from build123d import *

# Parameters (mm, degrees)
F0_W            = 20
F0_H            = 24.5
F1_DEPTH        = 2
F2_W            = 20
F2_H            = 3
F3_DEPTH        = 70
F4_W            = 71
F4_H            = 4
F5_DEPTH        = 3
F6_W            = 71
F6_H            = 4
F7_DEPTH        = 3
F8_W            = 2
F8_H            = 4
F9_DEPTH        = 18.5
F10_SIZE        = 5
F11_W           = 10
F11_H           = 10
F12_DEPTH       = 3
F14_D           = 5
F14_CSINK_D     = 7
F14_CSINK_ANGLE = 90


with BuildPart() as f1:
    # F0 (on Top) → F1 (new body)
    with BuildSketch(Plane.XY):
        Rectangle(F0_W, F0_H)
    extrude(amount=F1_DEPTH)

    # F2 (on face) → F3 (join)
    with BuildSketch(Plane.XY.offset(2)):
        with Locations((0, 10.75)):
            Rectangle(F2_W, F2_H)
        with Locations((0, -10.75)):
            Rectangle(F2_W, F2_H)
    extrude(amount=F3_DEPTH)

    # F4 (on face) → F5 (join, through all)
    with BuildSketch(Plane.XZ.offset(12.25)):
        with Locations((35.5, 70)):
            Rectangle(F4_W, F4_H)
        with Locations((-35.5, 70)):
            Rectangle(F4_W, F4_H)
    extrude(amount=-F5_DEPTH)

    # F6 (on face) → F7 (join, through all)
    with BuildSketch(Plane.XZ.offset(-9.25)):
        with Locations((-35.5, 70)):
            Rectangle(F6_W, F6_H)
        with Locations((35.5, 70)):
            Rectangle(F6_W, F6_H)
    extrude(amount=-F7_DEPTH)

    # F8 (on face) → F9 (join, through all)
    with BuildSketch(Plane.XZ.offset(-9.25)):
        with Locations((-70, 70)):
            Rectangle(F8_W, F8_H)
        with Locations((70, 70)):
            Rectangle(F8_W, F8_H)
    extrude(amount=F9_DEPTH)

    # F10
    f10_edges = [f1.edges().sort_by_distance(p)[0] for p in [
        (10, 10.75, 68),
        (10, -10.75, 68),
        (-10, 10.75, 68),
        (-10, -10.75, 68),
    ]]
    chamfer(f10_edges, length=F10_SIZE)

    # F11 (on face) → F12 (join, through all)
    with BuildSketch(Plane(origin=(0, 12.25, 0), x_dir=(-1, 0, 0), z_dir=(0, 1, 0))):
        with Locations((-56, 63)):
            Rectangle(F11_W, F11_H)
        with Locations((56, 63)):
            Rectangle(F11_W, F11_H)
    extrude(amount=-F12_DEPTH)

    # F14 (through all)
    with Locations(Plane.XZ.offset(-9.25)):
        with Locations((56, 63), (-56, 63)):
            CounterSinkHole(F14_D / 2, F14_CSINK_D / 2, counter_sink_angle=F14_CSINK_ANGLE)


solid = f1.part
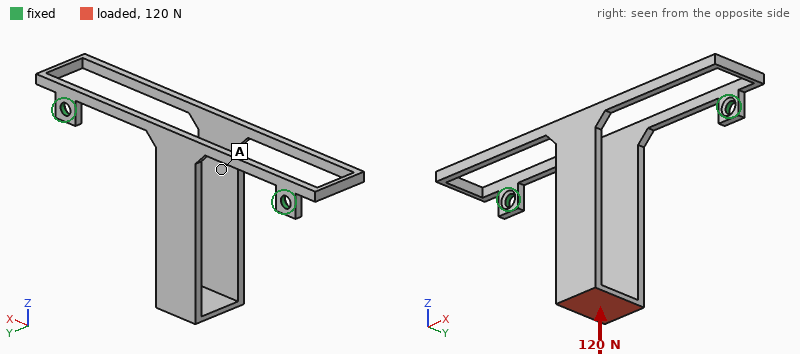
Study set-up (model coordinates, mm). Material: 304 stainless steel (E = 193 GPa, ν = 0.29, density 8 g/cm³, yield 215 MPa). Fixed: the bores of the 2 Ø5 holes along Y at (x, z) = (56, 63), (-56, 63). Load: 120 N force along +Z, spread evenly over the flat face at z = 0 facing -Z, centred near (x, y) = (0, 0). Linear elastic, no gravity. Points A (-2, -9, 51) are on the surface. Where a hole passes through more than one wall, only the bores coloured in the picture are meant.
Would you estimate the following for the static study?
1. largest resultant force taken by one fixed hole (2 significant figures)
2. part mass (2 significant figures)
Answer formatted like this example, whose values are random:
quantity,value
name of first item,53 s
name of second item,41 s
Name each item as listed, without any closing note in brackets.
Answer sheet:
quantity,value
largest resultant force taken by one fixed hole,60 N
part mass,110 g
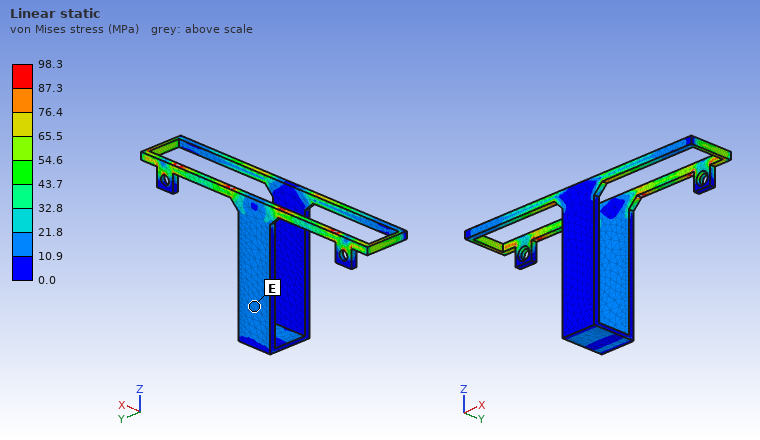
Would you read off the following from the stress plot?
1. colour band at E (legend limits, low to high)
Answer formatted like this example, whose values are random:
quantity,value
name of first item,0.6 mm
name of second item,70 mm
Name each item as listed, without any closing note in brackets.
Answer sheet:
quantity,value
colour band at E,10.9 to 21.8 MPa
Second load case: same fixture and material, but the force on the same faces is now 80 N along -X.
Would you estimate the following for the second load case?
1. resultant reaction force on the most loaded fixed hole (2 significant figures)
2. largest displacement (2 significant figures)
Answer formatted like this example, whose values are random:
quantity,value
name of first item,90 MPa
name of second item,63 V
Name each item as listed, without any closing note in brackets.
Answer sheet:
quantity,value
resultant reaction force on the most loaded fixed hole,78 N
largest displacement,0.29 mm
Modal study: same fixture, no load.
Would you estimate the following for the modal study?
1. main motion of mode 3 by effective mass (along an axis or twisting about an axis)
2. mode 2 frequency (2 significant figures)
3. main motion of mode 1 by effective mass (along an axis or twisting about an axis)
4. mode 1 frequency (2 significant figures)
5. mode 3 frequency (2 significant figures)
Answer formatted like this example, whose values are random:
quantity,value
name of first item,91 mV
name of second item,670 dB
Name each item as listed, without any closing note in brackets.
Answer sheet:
quantity,value
main motion of mode 3 by effective mass,along X
mode 2 frequency,400 Hz
main motion of mode 1 by effective mass,along Y
mode 1 frequency,130 Hz
mode 3 frequency,480 Hz
